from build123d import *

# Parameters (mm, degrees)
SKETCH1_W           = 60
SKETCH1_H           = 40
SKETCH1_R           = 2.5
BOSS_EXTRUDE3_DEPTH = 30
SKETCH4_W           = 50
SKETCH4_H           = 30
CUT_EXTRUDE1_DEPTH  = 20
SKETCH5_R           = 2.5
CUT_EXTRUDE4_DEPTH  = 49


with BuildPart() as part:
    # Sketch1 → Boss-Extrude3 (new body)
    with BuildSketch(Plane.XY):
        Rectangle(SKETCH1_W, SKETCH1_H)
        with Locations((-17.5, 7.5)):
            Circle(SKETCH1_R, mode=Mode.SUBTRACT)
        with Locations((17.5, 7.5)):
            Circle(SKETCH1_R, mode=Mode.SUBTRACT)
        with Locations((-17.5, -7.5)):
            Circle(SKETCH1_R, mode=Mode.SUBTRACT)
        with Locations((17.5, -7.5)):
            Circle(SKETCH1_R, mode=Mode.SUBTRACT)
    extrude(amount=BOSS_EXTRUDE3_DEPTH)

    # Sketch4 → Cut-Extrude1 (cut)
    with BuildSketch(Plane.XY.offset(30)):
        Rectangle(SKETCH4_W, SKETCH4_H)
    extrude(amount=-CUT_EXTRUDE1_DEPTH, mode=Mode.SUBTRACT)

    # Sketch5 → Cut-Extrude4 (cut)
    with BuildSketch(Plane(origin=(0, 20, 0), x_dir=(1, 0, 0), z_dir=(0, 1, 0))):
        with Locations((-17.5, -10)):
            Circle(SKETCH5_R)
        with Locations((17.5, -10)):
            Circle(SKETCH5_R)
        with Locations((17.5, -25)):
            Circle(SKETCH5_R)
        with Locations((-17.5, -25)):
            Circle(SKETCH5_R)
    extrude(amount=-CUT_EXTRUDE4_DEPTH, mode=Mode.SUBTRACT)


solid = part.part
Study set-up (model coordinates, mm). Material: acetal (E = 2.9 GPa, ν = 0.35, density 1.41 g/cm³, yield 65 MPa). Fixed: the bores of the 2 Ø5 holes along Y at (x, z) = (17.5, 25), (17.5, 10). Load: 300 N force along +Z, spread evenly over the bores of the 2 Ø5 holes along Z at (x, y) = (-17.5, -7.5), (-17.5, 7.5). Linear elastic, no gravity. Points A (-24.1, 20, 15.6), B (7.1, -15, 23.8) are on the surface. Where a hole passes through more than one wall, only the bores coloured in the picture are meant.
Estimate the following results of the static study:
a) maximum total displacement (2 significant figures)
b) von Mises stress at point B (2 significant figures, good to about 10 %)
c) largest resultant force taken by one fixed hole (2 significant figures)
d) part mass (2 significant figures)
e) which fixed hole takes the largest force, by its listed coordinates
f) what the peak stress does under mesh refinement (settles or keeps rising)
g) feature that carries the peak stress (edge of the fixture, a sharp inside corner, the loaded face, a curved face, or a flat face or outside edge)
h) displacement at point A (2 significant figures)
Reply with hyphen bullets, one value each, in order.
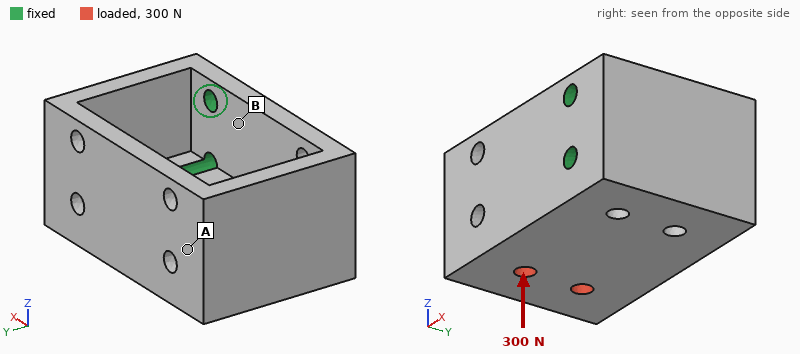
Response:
- 0.82 mm
- 7.2 MPa
- 590 N
- 56 g
- (17.5, 10)
- keeps rising
- edge of the fixture
- 0.68 mm
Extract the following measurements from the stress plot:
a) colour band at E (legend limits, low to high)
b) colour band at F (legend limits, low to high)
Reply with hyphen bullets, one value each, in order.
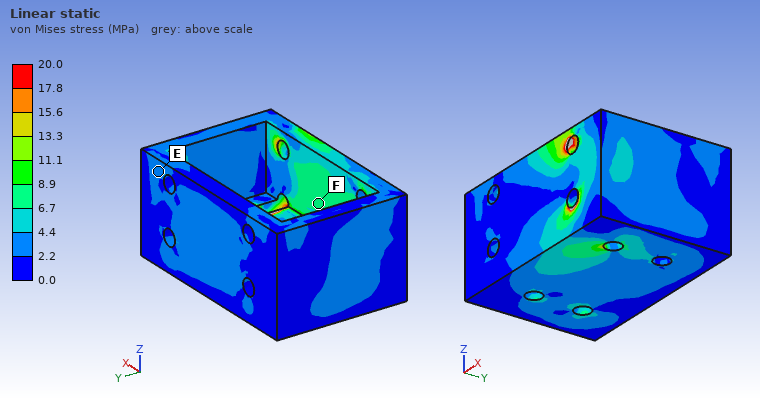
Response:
- 2.2 to 4.4 MPa
- 6.7 to 8.9 MPa
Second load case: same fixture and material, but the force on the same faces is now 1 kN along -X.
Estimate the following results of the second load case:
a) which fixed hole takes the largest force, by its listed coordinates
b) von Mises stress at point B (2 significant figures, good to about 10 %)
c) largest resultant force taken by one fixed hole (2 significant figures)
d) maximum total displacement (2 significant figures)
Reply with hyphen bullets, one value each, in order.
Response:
- (17.5, 10)
- 4.3 MPa
- 1.2 kN
- 0.81 mm
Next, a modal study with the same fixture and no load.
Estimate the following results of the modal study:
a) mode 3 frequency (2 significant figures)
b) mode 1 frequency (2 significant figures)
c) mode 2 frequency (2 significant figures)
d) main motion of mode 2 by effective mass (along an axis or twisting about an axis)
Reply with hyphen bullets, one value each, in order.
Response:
- 1600 Hz
- 650 Hz
- 680 Hz
- along Z
